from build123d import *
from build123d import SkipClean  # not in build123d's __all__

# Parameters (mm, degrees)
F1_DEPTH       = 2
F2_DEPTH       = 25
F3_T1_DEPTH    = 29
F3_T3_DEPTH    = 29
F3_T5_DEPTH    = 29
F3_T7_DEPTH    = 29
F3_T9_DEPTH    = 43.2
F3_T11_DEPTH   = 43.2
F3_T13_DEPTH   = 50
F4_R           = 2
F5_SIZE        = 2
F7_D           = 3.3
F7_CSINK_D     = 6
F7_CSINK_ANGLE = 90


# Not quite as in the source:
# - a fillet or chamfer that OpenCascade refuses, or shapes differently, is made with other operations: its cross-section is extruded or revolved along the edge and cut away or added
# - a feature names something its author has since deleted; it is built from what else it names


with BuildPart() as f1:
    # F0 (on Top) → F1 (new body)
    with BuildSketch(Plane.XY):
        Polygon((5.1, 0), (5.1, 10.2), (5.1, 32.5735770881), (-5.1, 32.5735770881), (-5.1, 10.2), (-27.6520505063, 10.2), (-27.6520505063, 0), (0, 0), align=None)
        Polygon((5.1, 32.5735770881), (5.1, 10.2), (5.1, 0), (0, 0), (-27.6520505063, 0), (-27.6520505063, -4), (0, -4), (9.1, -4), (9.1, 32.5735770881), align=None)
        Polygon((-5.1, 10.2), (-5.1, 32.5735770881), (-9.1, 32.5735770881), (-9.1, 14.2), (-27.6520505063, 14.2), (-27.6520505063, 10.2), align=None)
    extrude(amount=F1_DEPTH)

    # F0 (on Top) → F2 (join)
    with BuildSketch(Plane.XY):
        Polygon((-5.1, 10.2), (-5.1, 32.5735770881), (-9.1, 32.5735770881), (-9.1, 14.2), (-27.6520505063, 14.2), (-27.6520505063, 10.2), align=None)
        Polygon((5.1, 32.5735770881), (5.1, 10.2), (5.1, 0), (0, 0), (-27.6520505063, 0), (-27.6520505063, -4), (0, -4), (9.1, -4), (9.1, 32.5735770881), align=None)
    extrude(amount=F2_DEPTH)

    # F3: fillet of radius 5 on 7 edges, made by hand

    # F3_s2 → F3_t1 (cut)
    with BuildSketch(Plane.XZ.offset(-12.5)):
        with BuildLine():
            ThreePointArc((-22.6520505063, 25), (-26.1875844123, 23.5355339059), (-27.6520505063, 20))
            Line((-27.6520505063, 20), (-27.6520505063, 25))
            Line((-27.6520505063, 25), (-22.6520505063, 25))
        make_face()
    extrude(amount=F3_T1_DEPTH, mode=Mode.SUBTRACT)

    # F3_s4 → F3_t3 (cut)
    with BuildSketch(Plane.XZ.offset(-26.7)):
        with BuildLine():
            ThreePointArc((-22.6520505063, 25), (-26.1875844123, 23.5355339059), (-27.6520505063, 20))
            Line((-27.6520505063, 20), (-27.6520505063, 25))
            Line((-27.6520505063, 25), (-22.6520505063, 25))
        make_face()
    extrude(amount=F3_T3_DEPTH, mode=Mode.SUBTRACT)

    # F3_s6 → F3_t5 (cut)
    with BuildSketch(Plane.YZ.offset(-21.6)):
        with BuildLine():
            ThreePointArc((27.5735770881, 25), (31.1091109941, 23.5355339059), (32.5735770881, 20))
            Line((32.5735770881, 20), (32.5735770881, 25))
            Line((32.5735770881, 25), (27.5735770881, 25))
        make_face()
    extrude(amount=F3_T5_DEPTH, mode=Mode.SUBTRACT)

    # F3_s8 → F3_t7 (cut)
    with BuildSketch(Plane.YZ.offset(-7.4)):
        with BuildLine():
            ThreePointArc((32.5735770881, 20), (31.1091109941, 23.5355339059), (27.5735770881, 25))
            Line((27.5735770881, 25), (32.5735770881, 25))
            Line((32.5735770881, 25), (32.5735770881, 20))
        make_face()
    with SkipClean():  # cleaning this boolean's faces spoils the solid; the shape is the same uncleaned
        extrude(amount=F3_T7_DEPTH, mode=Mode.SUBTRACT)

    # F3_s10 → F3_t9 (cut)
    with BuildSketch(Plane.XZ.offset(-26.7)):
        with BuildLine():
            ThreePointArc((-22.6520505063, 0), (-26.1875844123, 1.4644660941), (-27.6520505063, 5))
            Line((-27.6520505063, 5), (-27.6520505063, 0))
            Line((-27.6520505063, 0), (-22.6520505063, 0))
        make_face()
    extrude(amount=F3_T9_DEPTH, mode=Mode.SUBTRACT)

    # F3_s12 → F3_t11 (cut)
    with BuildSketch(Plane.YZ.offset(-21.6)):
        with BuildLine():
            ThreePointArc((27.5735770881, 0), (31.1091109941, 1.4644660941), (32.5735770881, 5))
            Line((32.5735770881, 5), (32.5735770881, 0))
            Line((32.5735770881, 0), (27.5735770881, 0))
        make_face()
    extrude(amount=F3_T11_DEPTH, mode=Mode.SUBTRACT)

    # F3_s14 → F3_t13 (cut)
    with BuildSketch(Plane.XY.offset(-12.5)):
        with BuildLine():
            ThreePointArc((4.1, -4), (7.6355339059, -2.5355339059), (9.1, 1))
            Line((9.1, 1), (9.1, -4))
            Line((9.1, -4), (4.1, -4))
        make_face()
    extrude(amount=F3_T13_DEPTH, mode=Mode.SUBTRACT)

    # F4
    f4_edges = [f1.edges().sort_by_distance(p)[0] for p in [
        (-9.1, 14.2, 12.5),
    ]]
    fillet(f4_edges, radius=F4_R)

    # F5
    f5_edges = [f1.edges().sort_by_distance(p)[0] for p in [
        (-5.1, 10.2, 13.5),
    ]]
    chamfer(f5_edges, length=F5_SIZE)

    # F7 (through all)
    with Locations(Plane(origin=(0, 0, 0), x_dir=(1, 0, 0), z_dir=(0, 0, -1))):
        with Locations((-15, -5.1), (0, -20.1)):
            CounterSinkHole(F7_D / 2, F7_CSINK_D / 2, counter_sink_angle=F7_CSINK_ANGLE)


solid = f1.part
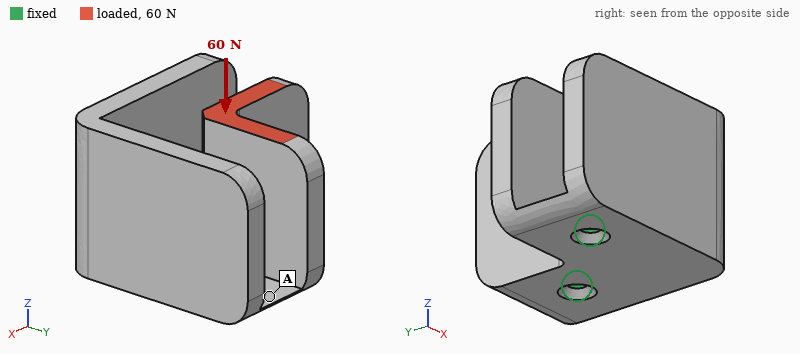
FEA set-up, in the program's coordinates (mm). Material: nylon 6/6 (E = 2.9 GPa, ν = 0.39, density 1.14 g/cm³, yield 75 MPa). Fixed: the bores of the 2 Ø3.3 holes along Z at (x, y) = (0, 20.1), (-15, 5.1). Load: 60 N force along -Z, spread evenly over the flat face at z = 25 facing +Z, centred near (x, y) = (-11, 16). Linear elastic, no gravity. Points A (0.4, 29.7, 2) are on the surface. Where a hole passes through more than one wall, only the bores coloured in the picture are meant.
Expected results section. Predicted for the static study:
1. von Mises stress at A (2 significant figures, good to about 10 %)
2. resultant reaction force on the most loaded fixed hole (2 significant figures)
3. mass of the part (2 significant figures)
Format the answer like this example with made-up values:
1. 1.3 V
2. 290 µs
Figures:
1. 2.6 MPa
2. 30 N
3. 13 g
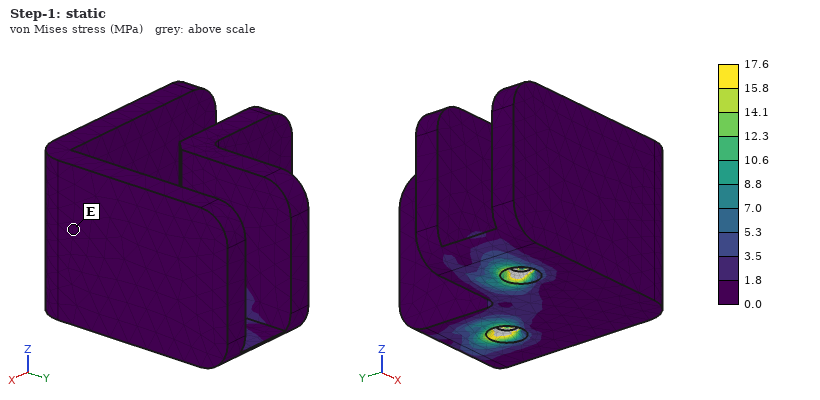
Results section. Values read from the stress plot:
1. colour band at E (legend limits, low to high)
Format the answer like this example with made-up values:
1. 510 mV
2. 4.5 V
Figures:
1. 0.0 to 1.8 MPa
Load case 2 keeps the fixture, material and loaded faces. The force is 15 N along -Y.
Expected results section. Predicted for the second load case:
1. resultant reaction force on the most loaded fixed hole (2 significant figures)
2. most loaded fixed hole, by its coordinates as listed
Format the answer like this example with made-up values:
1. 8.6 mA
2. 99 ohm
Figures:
1. 19 N
2. (0, 20.1)
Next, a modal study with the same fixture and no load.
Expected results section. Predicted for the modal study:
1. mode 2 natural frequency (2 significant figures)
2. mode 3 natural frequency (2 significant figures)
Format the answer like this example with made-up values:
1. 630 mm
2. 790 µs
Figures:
1. 810 Hz
2. 870 Hz
